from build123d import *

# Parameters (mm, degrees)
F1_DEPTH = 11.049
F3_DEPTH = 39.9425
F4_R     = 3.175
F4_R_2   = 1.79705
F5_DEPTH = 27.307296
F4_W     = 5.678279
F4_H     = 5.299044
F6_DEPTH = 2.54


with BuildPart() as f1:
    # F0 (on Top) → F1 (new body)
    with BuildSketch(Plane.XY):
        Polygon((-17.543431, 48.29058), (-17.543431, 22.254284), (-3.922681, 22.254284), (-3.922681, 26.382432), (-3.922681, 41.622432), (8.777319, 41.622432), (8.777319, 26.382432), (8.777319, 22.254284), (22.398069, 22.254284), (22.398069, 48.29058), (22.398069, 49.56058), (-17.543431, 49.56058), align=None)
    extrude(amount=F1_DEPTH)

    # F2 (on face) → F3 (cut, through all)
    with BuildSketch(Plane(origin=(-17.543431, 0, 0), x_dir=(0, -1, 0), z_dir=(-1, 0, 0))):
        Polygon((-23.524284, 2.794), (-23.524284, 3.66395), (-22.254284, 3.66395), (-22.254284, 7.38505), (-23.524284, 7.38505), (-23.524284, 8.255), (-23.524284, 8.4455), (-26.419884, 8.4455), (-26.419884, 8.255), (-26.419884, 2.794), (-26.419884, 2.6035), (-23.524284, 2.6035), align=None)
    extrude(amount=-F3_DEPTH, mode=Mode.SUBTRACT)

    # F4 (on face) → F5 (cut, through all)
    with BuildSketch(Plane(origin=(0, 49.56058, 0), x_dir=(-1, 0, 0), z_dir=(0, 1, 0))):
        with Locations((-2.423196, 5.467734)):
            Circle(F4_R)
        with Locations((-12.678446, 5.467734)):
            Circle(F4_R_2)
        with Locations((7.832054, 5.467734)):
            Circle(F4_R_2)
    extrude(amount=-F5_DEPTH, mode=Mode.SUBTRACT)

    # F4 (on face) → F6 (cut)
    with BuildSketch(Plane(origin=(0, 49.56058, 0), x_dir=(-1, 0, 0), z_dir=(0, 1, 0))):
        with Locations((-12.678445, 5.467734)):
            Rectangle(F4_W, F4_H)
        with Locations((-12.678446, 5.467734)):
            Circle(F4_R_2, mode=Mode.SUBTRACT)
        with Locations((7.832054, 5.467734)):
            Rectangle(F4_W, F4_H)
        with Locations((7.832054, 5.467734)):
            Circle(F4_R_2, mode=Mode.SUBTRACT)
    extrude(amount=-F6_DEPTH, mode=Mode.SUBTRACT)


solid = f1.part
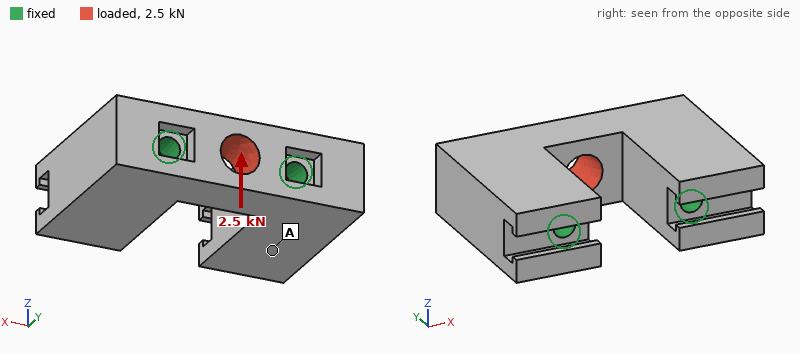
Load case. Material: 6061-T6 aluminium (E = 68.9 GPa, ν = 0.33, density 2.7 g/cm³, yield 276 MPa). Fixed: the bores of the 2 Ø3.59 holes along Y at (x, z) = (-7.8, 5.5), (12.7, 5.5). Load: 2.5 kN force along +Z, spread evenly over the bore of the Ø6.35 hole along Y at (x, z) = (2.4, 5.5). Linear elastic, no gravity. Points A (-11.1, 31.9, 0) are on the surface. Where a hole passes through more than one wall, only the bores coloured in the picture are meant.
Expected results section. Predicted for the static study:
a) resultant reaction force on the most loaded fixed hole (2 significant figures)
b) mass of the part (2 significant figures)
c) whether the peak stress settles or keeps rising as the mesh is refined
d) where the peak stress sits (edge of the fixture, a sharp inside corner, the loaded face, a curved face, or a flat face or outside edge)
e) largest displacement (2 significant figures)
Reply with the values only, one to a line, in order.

1.3 kN
21 g
keeps rising
edge of the fixture
11 µm
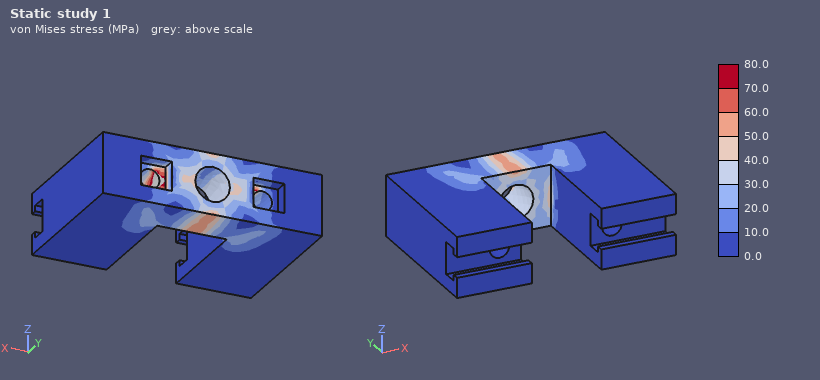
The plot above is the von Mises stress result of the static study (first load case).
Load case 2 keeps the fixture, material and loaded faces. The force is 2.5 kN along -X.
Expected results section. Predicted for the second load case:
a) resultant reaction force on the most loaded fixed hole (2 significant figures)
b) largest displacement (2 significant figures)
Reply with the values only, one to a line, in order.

1.3 kN
2.8 µm
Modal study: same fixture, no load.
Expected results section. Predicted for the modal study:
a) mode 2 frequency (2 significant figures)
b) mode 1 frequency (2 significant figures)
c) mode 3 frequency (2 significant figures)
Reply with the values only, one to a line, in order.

38 kHz
38 kHz
47 kHz
